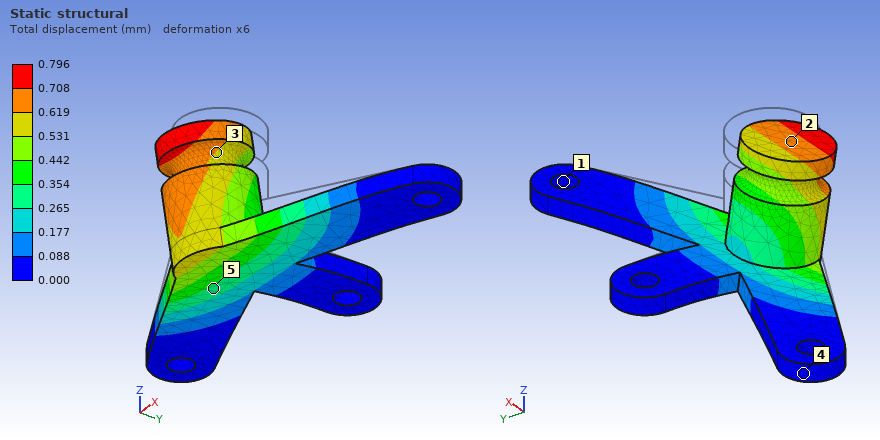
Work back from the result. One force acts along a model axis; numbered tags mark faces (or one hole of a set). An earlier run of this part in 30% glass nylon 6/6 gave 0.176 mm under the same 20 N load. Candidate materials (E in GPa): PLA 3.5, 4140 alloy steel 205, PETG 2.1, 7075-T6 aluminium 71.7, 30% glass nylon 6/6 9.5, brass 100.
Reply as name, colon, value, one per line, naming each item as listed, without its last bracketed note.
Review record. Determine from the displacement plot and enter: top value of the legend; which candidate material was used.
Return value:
top value of the legend: 0.796 mm
which candidate material was used: PETG
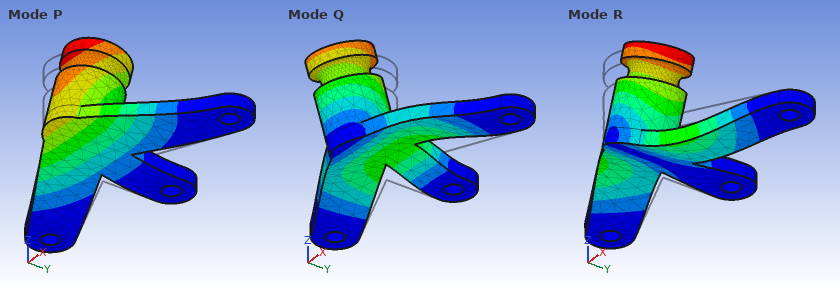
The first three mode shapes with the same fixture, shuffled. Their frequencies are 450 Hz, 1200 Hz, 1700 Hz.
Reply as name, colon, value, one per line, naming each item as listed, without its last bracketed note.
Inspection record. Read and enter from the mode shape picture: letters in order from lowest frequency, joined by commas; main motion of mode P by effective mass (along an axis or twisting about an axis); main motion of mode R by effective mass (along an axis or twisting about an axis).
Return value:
letters in order from lowest frequency, joined by commas: P, R, Q
main motion of mode P by effective mass: along Z
main motion of mode R by effective mass: along X
